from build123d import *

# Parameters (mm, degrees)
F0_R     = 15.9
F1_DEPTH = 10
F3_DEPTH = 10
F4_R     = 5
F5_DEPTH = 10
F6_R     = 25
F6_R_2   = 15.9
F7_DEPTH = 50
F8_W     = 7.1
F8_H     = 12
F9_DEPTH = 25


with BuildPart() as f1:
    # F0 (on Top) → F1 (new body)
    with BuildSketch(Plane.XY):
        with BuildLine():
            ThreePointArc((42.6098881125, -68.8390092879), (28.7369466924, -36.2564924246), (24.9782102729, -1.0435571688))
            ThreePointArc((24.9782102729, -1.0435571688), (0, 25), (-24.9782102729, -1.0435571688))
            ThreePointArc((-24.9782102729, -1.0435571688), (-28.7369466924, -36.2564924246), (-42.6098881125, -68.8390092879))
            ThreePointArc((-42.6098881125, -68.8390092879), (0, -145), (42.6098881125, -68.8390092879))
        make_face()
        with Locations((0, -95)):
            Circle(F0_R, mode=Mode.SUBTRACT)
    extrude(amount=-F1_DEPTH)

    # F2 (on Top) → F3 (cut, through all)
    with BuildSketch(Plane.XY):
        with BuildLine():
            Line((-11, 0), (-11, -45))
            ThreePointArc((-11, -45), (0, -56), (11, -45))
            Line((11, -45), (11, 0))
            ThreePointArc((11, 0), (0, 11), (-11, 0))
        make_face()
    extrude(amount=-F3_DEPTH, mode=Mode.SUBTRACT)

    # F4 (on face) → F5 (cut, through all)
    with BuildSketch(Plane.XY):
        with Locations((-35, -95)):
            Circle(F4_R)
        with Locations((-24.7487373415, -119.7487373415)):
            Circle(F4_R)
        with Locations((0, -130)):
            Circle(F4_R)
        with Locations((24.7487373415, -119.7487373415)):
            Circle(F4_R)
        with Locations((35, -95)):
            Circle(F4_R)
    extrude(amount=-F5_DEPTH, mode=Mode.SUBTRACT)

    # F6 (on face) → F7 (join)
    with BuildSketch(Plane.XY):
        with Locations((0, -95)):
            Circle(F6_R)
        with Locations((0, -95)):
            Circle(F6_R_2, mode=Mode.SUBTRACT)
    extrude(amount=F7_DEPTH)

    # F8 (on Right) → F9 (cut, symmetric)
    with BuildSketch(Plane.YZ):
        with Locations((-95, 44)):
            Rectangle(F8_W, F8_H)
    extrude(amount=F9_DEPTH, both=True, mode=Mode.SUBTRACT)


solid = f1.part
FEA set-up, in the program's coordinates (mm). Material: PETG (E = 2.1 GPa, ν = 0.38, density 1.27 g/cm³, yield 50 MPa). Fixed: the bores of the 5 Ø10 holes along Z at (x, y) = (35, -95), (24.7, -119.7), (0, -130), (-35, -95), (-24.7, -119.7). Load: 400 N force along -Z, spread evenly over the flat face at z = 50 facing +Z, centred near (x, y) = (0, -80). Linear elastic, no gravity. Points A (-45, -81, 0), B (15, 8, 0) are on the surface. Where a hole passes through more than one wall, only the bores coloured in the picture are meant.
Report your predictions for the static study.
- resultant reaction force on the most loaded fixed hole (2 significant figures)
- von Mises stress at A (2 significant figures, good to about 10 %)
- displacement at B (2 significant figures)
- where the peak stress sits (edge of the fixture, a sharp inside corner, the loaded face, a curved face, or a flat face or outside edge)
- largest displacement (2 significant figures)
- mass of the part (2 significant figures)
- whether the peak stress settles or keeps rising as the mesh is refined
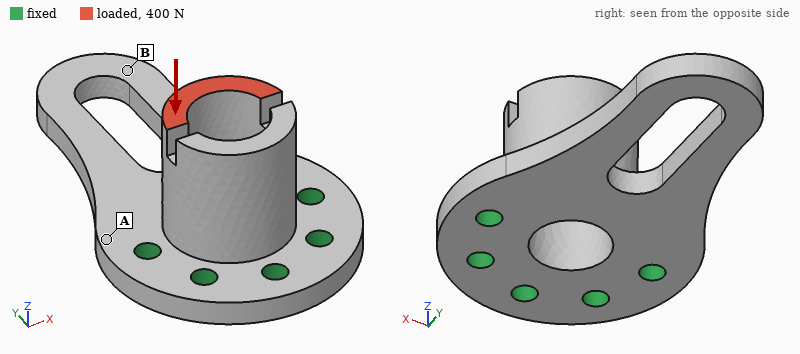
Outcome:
250 N
1.1 MPa
0.24 mm
edge of the fixture
0.28 mm
190 g
keeps rising
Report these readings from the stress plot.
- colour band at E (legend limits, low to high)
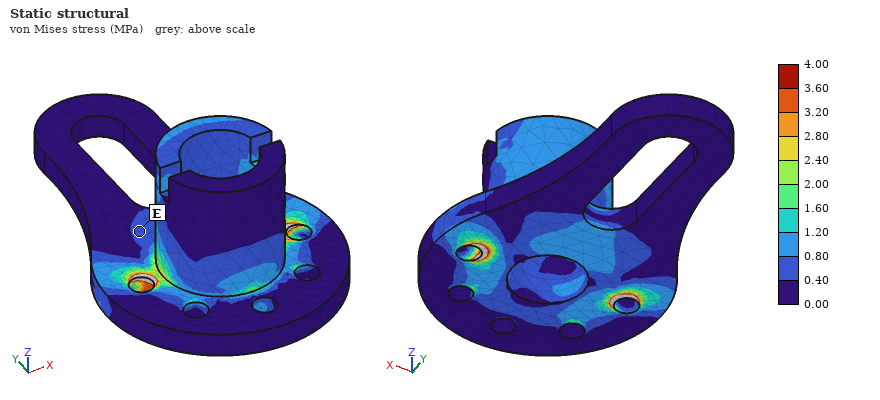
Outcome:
0.40 to 0.80 MPa
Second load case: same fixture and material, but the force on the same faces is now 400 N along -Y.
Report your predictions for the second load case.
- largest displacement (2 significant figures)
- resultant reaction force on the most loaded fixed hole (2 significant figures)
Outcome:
0.59 mm
330 N
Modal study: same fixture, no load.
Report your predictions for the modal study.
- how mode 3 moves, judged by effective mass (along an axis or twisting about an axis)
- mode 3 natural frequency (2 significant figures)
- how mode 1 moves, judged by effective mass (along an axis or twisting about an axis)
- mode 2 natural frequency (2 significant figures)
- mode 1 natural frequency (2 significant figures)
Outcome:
along X
890 Hz
along Z
730 Hz
240 Hz
